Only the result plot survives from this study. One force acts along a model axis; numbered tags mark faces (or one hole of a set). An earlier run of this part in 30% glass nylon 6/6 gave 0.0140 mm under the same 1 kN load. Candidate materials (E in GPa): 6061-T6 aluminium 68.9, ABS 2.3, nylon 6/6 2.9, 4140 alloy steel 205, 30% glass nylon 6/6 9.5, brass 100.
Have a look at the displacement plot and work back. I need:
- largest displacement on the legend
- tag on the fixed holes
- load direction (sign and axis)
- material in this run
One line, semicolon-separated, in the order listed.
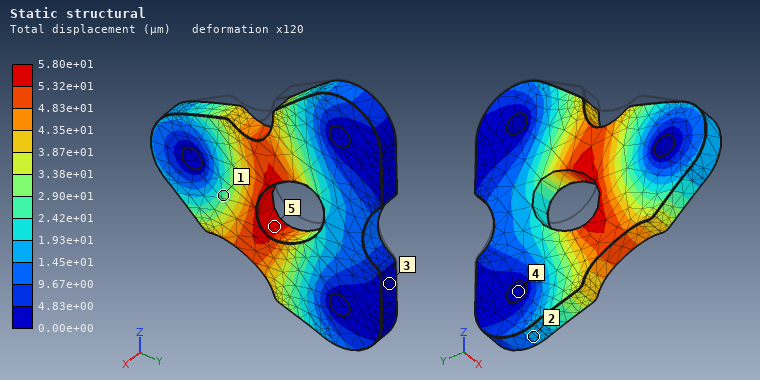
5.80e+01 µm; 4; -Z; ABS
